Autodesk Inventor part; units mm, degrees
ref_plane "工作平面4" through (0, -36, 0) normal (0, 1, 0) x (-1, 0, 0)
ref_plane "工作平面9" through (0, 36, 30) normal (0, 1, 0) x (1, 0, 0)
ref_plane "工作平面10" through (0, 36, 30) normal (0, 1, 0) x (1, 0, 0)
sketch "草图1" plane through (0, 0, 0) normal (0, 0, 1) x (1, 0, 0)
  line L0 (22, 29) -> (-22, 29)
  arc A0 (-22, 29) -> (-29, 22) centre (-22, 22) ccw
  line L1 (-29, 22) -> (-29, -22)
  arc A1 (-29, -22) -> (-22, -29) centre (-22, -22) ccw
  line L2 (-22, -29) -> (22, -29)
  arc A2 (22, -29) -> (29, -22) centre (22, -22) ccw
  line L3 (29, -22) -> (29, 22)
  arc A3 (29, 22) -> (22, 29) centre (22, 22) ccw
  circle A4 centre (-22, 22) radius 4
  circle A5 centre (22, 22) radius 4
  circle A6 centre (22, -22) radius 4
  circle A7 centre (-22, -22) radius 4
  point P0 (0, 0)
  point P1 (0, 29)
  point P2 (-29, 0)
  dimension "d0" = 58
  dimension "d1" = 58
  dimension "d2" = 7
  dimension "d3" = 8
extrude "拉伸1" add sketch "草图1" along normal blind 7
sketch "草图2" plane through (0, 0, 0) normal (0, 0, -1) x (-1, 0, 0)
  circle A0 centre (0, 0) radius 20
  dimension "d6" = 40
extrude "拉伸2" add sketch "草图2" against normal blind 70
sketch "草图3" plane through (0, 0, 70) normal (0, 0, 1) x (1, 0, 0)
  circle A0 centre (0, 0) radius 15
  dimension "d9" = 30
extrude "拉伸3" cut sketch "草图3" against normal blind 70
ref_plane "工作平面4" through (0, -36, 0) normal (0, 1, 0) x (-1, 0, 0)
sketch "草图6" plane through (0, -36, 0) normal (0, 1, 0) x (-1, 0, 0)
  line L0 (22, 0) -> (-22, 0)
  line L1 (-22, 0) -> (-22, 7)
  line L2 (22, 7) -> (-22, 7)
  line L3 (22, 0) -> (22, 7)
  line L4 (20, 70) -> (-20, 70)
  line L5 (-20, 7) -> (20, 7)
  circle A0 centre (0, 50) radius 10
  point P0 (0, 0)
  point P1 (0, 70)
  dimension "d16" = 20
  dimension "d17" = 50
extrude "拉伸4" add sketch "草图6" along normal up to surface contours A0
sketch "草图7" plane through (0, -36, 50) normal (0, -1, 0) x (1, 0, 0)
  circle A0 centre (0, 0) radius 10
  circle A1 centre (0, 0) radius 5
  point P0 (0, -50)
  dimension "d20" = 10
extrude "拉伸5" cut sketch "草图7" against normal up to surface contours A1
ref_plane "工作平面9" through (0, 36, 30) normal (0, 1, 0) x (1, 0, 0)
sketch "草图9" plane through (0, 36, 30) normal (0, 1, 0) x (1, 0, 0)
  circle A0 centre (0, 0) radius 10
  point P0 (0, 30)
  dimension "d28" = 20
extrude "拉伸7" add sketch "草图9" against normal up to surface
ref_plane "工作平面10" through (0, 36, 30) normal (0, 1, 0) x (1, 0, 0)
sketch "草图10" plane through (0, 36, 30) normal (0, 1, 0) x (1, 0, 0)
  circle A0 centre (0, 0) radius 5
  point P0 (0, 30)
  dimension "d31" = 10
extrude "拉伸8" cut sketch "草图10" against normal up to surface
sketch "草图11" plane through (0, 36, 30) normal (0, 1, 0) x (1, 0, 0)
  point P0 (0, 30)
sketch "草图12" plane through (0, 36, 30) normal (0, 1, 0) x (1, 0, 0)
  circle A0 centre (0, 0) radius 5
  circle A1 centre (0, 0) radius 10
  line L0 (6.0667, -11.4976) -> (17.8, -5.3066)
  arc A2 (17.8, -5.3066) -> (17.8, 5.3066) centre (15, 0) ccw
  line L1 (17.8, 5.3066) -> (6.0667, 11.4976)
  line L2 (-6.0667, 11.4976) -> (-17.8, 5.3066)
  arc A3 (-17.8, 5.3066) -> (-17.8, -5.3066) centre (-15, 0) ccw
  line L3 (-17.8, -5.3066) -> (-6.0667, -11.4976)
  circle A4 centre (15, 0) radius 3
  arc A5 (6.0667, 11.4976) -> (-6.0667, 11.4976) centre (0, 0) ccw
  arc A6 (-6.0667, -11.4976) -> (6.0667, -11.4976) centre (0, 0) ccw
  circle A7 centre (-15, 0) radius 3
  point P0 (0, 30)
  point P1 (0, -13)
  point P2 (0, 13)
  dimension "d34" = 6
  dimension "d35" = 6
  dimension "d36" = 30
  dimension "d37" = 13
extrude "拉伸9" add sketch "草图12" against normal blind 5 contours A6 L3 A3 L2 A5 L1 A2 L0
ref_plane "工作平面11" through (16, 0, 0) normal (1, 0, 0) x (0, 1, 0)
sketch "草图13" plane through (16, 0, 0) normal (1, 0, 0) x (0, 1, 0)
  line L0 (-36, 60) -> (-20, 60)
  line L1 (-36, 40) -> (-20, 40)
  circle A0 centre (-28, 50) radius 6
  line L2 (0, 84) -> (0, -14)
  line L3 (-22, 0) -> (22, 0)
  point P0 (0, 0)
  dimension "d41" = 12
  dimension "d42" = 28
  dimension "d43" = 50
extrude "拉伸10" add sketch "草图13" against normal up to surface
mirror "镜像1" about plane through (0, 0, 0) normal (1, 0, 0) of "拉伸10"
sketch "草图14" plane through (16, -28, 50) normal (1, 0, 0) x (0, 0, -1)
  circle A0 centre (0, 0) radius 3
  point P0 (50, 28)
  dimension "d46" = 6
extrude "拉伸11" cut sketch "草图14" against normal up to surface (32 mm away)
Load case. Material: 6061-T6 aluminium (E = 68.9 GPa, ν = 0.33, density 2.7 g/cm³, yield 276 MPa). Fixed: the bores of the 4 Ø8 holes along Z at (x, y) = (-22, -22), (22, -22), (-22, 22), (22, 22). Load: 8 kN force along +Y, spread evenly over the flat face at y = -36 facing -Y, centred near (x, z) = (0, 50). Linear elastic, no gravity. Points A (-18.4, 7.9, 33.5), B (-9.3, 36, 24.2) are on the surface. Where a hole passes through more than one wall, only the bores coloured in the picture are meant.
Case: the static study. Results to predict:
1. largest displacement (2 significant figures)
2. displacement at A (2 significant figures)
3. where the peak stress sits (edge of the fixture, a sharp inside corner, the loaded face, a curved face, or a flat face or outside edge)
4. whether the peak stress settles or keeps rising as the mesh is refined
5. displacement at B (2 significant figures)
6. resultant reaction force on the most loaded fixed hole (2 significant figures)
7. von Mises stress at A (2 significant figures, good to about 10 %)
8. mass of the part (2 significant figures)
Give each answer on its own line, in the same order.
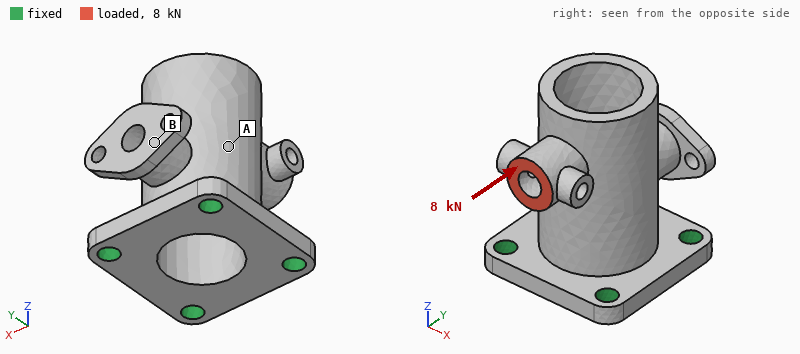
0.33 mm
0.12 mm
edge of the fixture
keeps rising
0.15 mm
5.6 kN
50 MPa
170 g
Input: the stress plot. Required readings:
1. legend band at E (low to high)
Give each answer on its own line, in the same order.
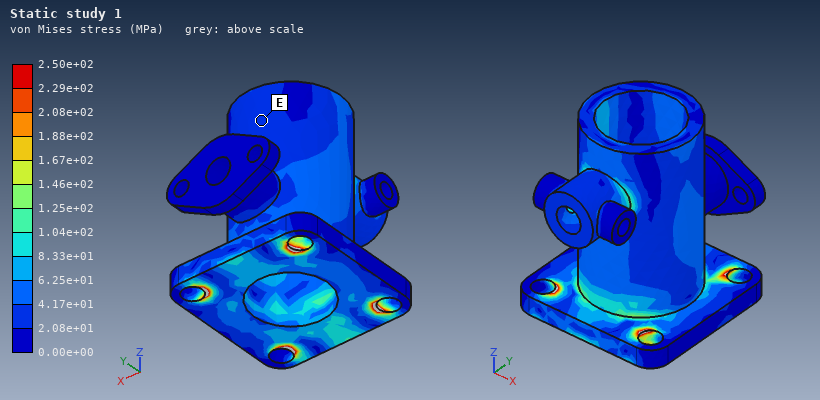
2.08e+01 to 4.17e+01 MPa
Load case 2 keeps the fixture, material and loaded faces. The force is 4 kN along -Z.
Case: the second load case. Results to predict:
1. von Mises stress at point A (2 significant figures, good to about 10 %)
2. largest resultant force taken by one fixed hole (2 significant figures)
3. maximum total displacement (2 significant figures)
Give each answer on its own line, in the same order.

23 MPa
3.1 kN
0.24 mm
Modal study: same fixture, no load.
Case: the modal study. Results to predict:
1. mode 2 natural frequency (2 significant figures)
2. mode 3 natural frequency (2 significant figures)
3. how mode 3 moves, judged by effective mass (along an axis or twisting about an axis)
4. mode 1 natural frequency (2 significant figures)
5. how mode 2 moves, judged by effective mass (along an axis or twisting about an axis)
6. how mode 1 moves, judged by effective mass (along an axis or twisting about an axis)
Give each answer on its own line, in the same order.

3400 Hz
7300 Hz
twisting about Z
3200 Hz
along X
along Y
